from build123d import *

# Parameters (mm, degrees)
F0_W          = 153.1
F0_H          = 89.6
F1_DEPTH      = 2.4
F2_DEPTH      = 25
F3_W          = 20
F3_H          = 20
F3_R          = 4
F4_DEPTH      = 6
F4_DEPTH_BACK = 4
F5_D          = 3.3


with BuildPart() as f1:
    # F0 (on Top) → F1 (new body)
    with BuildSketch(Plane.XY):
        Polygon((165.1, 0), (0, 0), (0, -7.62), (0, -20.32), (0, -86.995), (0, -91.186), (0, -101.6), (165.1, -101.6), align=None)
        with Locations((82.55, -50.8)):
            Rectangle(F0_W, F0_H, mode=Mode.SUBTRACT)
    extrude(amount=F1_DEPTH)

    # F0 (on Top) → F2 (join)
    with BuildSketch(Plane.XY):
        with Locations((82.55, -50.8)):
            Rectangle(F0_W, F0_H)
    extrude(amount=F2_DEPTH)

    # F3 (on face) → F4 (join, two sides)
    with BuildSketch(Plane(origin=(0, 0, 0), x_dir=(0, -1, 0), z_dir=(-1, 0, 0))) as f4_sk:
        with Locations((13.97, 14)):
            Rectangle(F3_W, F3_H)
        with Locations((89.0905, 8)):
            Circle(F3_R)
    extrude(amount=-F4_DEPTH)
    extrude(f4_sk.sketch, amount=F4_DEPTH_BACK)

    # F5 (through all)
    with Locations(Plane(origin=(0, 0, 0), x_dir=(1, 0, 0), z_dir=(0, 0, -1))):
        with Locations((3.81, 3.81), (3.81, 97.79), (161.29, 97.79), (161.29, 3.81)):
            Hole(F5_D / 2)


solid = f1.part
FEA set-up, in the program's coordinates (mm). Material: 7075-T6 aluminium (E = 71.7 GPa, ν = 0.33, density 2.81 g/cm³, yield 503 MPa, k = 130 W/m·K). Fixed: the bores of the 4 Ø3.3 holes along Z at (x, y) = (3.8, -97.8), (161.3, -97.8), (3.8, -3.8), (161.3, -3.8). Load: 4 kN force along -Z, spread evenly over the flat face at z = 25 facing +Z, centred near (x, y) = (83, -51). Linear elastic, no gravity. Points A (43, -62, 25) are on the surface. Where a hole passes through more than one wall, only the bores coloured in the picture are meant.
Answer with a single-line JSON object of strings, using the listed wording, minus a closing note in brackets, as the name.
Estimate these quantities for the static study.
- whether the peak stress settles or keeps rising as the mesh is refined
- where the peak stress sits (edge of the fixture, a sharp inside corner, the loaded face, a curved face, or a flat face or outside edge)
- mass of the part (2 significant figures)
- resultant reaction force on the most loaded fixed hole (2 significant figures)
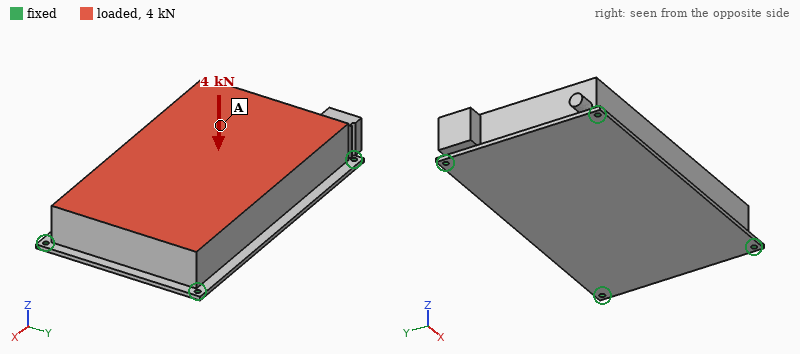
{"whether the peak stress settles or keeps rising as the mesh is refined": "keeps rising", "where the peak stress sits": "edge of the fixture", "mass of the part": "1000 g", "resultant reaction force on the most loaded fixed hole": "1.4 kN"}
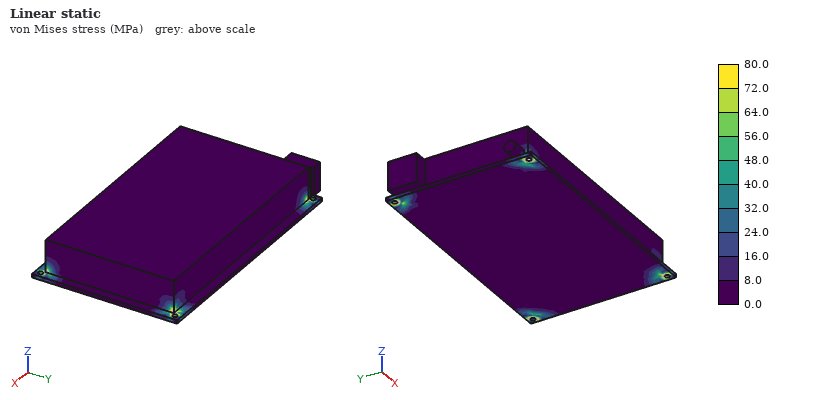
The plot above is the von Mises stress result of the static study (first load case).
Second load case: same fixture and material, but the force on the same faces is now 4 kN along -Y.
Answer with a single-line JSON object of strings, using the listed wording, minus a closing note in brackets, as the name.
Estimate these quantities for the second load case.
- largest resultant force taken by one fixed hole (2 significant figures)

{"largest resultant force taken by one fixed hole": "1.3 kN"}
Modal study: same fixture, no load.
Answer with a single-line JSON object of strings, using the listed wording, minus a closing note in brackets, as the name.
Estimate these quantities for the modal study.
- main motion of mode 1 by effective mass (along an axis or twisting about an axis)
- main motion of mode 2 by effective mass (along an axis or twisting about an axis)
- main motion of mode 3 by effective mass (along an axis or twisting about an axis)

{"main motion of mode 1 by effective mass": "along Z", "main motion of mode 2 by effective mass": "along Y", "main motion of mode 3 by effective mass": "twisting about Y"}
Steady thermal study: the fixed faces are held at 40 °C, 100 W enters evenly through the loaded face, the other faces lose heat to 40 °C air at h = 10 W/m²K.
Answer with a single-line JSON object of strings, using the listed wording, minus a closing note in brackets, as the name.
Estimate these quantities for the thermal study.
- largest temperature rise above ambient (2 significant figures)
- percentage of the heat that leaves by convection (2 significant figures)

{"largest temperature rise above ambient": "50 K", "percentage of the heat that leaves by convection": "15 %"}
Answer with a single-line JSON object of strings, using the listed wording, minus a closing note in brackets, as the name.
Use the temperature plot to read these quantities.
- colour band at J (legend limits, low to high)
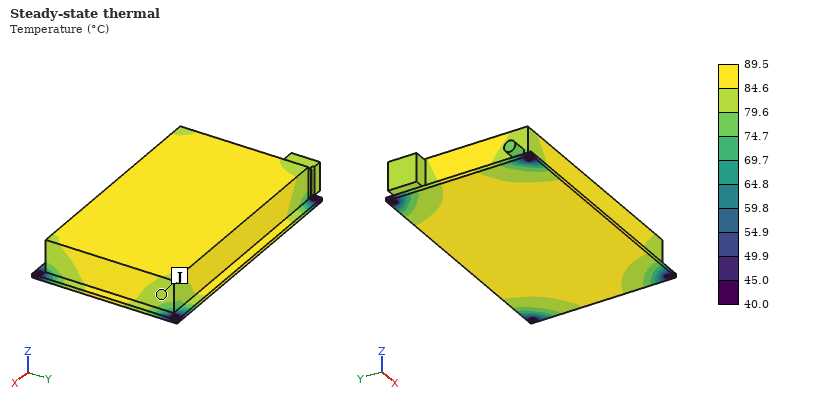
{"colour band at J": "79.6 to 84.6 °C"}
